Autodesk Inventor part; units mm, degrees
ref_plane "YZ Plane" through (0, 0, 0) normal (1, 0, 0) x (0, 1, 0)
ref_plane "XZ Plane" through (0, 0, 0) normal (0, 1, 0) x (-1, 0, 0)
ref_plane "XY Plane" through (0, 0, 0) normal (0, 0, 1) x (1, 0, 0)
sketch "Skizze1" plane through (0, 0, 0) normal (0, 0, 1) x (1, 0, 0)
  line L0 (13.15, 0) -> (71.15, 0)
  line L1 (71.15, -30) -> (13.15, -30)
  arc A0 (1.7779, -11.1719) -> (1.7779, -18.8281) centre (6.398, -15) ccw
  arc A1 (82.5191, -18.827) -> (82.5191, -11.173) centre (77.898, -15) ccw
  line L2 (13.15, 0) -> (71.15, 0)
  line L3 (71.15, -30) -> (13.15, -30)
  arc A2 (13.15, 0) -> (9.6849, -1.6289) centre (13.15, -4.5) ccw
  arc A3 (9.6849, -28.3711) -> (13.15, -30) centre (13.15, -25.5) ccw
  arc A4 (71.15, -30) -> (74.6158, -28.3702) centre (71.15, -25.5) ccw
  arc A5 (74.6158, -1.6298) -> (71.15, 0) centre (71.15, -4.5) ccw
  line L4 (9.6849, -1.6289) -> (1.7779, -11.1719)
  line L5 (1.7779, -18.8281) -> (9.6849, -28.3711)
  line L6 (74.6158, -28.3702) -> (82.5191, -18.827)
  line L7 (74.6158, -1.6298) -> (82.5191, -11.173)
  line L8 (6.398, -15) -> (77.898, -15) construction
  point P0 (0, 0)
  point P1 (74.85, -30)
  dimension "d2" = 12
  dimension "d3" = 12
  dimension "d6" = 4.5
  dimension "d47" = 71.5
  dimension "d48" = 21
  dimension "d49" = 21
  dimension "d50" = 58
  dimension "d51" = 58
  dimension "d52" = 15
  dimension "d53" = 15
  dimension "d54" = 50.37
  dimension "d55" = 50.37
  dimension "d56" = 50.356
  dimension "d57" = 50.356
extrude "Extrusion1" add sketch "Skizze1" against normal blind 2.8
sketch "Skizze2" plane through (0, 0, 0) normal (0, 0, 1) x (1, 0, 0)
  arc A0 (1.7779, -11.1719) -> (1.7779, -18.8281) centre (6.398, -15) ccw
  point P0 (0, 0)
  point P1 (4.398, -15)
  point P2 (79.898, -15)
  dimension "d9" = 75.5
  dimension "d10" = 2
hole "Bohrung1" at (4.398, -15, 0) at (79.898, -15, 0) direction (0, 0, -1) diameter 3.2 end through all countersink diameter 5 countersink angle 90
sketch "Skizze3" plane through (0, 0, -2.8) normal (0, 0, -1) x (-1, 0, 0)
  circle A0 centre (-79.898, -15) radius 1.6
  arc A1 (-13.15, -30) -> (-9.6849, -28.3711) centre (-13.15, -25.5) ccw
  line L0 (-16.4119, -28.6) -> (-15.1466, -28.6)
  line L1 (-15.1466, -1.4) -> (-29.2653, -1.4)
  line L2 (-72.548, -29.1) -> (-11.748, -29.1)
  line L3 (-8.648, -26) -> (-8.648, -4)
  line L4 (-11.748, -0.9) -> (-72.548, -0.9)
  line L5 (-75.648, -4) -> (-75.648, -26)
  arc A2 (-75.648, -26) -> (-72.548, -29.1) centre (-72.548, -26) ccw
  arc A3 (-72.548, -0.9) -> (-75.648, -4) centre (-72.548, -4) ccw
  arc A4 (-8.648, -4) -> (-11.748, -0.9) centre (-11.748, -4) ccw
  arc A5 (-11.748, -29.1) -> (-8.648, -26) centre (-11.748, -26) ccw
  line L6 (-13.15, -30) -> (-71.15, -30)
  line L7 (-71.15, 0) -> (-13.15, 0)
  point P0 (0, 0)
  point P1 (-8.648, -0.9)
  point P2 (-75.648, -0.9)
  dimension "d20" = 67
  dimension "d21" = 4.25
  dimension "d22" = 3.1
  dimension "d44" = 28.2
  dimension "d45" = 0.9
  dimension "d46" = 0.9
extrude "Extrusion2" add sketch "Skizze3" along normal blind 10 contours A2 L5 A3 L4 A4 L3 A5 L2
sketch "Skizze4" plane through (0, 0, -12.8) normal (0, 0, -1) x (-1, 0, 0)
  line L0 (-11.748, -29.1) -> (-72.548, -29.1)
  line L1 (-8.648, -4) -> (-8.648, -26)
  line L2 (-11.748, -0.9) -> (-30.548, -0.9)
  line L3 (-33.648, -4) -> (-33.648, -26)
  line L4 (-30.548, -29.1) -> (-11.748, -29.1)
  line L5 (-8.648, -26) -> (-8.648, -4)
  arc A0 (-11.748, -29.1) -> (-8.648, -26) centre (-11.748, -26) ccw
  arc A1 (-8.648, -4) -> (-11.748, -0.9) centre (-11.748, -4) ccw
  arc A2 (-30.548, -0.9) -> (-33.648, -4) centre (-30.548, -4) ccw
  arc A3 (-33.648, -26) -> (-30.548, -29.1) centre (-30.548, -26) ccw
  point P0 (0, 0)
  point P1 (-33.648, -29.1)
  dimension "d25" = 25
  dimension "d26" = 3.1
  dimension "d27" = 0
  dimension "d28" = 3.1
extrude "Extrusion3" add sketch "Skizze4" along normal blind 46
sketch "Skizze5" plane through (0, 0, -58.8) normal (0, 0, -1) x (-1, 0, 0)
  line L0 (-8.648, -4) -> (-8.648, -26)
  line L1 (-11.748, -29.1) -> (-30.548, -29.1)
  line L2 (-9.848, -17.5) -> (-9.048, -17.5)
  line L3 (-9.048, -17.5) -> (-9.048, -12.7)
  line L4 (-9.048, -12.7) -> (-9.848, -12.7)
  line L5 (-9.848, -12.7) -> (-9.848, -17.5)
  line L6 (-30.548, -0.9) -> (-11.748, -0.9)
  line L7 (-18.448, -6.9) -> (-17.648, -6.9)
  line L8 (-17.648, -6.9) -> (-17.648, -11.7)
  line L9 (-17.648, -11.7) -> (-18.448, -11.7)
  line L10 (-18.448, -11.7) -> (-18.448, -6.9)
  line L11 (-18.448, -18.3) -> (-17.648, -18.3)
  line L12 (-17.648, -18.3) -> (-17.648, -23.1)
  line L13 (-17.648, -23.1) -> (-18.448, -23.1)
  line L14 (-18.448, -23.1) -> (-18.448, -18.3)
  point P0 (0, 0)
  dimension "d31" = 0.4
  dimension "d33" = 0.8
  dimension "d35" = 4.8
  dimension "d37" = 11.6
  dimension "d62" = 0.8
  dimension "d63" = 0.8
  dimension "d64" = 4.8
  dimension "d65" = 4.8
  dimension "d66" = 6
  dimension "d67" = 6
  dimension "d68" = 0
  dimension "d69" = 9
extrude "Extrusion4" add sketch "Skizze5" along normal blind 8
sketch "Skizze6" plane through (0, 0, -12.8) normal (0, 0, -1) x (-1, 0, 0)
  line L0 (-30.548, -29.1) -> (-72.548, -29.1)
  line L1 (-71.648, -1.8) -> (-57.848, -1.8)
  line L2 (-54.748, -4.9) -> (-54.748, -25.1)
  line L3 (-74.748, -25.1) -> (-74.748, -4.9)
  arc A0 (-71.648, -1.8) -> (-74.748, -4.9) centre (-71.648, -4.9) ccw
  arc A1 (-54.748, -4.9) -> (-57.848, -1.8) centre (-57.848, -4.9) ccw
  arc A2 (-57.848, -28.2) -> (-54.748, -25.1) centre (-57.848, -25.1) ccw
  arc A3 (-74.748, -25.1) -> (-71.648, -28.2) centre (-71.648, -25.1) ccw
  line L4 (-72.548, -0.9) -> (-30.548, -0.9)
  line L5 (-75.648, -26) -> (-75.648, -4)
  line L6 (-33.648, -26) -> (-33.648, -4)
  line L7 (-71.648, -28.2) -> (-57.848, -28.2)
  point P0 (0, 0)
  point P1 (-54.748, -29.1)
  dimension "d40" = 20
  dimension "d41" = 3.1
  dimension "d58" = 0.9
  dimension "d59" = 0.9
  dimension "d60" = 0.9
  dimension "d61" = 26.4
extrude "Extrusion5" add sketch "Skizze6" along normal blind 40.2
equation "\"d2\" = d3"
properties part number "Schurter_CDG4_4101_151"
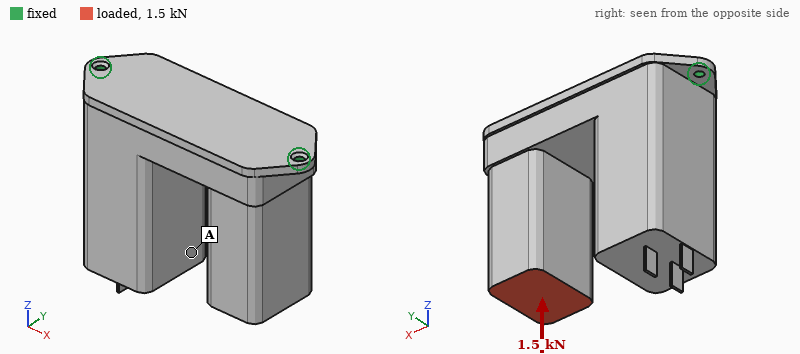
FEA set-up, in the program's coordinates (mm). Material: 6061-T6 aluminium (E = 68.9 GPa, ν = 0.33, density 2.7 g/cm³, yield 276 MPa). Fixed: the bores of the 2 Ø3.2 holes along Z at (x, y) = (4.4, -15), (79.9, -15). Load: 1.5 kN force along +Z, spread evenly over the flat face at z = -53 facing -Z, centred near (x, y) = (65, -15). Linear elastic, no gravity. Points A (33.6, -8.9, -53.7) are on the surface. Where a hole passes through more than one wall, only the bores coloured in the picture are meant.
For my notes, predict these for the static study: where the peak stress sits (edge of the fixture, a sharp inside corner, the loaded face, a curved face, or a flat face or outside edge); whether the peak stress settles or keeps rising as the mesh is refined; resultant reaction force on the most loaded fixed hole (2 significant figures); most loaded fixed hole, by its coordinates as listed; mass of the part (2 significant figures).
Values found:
edge of the fixture
keeps rising
1.3 kN
(79.9, -15)
210 g
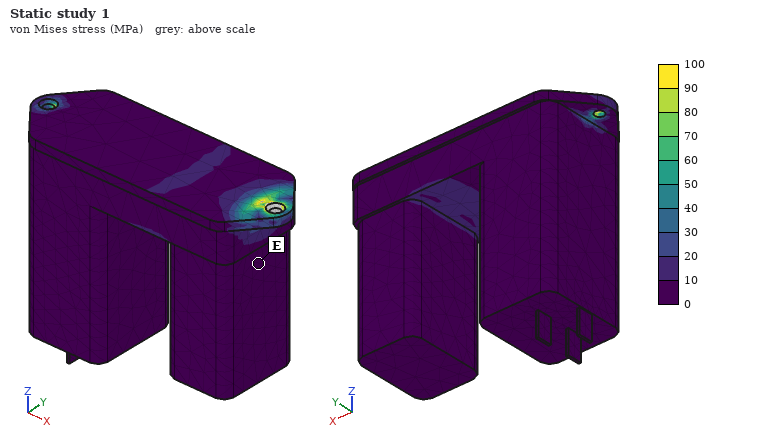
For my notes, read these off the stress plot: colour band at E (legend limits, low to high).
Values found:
0 to 10 MPa
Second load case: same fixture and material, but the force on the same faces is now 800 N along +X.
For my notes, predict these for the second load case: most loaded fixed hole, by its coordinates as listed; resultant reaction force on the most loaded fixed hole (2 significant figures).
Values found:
(4.4, -15)
1.2 kN
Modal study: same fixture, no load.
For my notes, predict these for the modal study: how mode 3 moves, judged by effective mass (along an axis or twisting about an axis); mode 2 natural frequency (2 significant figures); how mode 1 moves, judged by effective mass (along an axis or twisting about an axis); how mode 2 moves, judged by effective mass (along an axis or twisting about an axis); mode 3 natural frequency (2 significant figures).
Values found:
twisting about Z
2300 Hz
along Y
along Z
2800 Hz
